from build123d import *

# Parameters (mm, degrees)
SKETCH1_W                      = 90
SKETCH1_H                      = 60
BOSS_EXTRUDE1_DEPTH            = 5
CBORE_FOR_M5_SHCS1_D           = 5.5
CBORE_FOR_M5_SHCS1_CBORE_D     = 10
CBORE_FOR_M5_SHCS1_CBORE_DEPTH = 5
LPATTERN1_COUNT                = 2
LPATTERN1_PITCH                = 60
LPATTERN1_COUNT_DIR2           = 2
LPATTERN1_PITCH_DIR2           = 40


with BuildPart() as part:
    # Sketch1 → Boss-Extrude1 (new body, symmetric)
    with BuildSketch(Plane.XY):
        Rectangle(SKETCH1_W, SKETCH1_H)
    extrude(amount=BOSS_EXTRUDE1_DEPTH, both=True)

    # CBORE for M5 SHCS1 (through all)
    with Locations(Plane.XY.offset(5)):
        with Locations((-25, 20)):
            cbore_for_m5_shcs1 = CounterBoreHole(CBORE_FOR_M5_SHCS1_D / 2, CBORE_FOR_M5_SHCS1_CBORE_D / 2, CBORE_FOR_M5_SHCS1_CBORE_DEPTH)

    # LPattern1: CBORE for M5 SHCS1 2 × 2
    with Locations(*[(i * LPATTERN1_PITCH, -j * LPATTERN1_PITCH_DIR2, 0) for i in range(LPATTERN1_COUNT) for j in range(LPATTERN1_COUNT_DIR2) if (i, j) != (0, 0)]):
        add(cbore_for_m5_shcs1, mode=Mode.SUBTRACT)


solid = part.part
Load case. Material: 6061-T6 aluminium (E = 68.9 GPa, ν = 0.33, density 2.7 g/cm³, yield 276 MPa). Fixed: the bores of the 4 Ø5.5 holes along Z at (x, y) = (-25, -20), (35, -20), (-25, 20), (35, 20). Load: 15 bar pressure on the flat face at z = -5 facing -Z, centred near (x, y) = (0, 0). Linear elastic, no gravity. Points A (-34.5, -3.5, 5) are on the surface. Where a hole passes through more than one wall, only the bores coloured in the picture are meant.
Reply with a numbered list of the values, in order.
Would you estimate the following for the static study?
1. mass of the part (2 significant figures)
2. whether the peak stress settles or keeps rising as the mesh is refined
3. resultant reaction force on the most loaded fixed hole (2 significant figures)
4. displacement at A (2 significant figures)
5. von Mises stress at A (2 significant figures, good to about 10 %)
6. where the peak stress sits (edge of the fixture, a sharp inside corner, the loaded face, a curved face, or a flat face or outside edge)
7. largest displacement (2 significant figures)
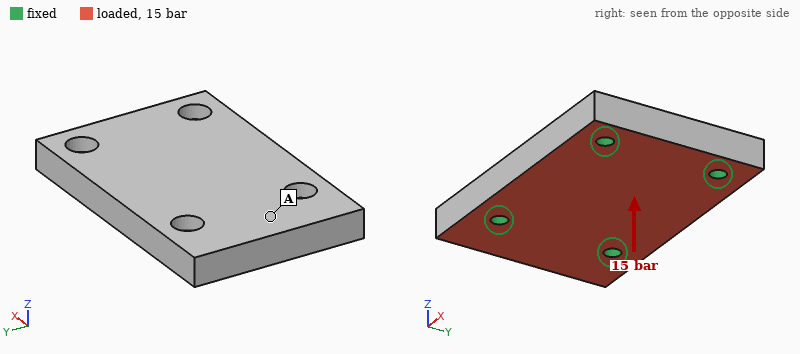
1. 140 g
2. keeps rising
3. 2.4 kN
4. 8.0 µm
5. 12 MPa
6. edge of the fixture
7. 20 µm
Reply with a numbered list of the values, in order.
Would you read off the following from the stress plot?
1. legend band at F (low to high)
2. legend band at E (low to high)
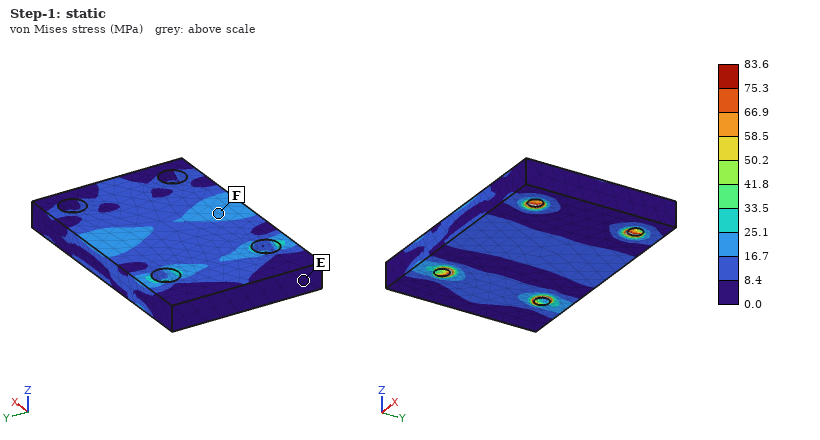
1. 16.7 to 25.1 MPa
2. 0.0 to 8.4 MPa
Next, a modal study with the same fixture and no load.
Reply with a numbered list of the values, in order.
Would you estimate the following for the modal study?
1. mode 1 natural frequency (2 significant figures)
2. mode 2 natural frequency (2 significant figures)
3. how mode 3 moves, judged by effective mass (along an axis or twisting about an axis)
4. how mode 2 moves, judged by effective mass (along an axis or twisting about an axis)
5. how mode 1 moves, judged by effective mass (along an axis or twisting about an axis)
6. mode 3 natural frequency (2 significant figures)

1. 8400 Hz
2. 11 kHz
3. twisting about X
4. along Z
5. along Z
6. 12 kHz
